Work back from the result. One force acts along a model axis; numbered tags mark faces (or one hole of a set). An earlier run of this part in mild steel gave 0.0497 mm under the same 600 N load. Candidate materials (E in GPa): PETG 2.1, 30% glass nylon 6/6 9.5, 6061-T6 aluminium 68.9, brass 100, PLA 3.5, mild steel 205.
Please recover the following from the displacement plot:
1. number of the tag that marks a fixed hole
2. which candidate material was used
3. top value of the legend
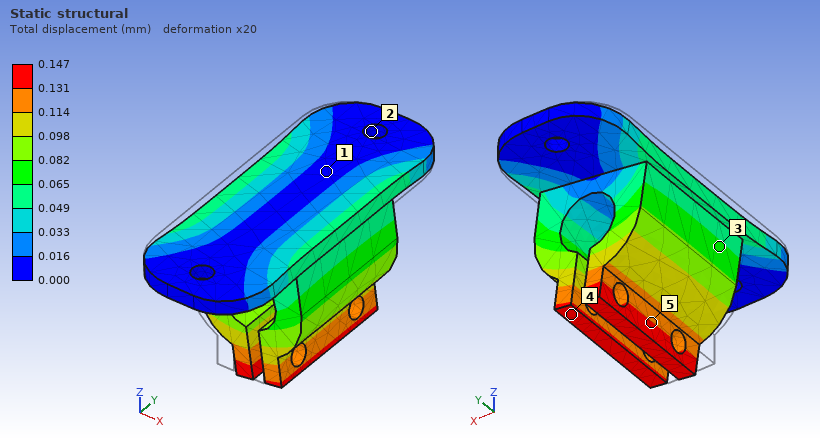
2
6061-T6 aluminium
0.147 mm
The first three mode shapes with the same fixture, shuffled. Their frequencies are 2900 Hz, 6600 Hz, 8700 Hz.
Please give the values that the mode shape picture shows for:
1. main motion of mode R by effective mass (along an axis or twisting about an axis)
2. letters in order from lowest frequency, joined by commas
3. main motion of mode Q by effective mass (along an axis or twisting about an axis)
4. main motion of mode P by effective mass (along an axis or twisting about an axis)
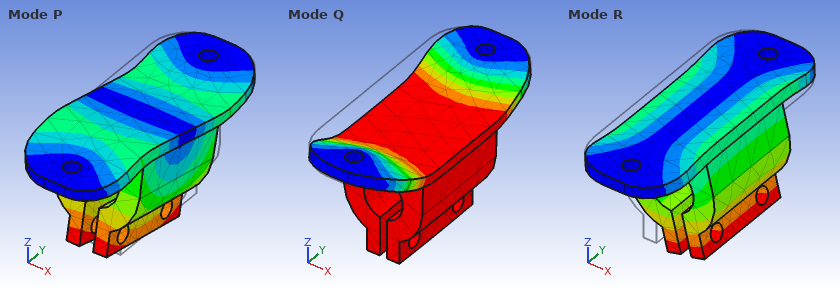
along X
R, Q, P
along Z
along Y
